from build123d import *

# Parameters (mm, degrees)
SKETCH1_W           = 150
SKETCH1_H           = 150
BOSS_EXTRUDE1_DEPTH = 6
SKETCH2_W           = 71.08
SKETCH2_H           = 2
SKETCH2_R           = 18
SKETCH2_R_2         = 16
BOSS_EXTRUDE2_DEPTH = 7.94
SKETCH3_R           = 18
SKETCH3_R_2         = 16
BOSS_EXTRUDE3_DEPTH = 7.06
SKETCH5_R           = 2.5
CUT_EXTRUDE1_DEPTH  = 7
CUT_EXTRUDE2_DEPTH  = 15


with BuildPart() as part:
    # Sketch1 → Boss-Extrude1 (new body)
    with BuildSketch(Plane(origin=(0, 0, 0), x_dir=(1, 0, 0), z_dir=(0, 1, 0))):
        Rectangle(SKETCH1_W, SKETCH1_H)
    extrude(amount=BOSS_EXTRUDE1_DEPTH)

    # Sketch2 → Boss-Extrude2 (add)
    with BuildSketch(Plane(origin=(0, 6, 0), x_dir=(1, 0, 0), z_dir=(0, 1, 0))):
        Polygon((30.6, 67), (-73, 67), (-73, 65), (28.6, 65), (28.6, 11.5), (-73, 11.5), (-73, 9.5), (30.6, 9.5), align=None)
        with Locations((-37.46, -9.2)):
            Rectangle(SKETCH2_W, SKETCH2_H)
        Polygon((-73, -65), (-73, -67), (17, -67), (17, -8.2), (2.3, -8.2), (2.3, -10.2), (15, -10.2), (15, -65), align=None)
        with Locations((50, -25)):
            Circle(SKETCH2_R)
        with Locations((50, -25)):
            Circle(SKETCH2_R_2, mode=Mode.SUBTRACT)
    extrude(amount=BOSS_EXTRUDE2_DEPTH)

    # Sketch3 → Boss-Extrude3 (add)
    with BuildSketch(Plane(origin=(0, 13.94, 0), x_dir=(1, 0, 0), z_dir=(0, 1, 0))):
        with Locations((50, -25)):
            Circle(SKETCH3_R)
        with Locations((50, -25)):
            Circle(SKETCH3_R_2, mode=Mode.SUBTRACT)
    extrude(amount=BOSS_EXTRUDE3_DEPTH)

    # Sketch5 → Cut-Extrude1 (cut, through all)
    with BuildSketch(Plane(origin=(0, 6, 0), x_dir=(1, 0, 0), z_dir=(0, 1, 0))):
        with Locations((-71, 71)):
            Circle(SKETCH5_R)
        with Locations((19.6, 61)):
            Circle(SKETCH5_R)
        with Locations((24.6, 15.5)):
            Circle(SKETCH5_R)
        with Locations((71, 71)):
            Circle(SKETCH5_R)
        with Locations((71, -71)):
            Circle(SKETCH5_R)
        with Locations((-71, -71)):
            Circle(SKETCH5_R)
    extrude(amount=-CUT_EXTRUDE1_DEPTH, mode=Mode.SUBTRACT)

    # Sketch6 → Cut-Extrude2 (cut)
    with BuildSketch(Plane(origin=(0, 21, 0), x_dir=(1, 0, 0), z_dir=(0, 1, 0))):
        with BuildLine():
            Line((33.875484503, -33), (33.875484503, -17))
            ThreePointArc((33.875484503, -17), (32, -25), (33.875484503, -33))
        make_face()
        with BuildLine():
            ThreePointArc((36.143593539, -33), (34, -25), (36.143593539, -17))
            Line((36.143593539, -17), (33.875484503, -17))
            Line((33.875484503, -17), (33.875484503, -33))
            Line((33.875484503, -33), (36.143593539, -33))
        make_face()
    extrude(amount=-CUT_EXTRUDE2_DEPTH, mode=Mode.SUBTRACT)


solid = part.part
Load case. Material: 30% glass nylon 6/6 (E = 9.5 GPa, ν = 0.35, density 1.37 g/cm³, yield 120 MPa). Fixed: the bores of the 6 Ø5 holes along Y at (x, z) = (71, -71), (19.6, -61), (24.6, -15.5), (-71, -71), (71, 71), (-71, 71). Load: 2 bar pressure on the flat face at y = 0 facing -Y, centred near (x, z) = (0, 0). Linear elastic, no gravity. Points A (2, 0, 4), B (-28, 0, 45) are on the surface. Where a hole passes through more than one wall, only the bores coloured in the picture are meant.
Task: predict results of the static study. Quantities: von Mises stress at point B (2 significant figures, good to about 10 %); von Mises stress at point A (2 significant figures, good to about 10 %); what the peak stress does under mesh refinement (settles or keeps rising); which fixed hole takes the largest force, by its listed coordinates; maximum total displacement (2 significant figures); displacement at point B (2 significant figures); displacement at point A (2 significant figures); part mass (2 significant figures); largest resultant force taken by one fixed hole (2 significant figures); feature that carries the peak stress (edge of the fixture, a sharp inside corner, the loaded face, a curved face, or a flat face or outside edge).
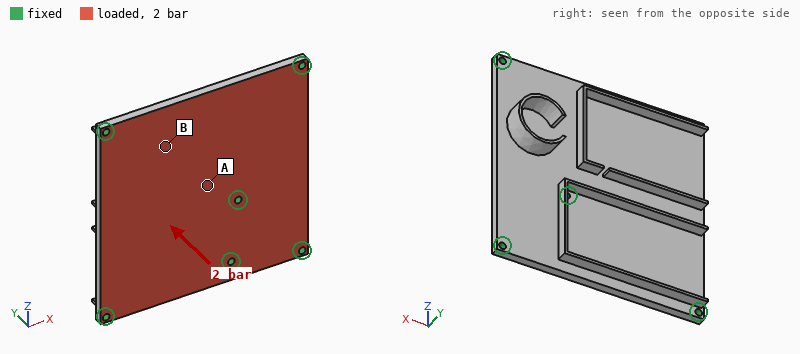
23 MPa
11 MPa
keeps rising
(24.6, -15.5)
1.6 mm
1.0 mm
0.61 mm
200 g
1.9 kN
edge of the fixture
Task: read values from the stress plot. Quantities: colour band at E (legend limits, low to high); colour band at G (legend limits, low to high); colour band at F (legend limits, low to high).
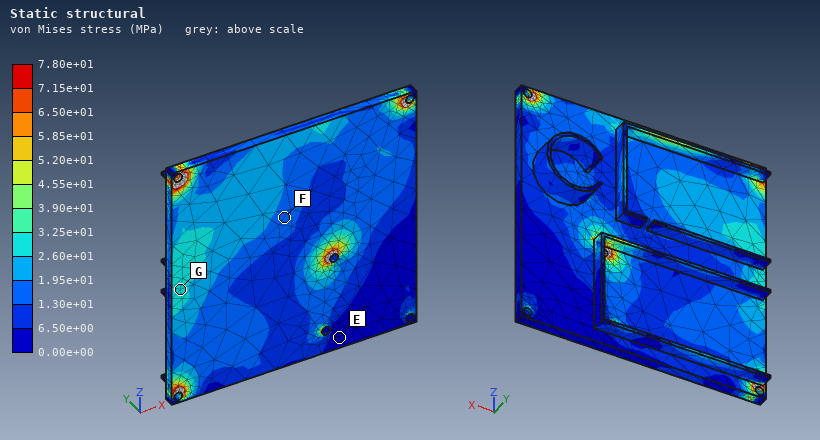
0.00e+00 to 6.50e+00 MPa
2.60e+01 to 3.25e+01 MPa
1.30e+01 to 1.95e+01 MPa
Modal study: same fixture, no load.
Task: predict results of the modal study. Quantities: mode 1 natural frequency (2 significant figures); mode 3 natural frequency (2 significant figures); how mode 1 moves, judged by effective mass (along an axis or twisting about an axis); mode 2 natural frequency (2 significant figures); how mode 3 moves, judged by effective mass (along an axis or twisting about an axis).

750 Hz
1300 Hz
along Y
940 Hz
along Y
